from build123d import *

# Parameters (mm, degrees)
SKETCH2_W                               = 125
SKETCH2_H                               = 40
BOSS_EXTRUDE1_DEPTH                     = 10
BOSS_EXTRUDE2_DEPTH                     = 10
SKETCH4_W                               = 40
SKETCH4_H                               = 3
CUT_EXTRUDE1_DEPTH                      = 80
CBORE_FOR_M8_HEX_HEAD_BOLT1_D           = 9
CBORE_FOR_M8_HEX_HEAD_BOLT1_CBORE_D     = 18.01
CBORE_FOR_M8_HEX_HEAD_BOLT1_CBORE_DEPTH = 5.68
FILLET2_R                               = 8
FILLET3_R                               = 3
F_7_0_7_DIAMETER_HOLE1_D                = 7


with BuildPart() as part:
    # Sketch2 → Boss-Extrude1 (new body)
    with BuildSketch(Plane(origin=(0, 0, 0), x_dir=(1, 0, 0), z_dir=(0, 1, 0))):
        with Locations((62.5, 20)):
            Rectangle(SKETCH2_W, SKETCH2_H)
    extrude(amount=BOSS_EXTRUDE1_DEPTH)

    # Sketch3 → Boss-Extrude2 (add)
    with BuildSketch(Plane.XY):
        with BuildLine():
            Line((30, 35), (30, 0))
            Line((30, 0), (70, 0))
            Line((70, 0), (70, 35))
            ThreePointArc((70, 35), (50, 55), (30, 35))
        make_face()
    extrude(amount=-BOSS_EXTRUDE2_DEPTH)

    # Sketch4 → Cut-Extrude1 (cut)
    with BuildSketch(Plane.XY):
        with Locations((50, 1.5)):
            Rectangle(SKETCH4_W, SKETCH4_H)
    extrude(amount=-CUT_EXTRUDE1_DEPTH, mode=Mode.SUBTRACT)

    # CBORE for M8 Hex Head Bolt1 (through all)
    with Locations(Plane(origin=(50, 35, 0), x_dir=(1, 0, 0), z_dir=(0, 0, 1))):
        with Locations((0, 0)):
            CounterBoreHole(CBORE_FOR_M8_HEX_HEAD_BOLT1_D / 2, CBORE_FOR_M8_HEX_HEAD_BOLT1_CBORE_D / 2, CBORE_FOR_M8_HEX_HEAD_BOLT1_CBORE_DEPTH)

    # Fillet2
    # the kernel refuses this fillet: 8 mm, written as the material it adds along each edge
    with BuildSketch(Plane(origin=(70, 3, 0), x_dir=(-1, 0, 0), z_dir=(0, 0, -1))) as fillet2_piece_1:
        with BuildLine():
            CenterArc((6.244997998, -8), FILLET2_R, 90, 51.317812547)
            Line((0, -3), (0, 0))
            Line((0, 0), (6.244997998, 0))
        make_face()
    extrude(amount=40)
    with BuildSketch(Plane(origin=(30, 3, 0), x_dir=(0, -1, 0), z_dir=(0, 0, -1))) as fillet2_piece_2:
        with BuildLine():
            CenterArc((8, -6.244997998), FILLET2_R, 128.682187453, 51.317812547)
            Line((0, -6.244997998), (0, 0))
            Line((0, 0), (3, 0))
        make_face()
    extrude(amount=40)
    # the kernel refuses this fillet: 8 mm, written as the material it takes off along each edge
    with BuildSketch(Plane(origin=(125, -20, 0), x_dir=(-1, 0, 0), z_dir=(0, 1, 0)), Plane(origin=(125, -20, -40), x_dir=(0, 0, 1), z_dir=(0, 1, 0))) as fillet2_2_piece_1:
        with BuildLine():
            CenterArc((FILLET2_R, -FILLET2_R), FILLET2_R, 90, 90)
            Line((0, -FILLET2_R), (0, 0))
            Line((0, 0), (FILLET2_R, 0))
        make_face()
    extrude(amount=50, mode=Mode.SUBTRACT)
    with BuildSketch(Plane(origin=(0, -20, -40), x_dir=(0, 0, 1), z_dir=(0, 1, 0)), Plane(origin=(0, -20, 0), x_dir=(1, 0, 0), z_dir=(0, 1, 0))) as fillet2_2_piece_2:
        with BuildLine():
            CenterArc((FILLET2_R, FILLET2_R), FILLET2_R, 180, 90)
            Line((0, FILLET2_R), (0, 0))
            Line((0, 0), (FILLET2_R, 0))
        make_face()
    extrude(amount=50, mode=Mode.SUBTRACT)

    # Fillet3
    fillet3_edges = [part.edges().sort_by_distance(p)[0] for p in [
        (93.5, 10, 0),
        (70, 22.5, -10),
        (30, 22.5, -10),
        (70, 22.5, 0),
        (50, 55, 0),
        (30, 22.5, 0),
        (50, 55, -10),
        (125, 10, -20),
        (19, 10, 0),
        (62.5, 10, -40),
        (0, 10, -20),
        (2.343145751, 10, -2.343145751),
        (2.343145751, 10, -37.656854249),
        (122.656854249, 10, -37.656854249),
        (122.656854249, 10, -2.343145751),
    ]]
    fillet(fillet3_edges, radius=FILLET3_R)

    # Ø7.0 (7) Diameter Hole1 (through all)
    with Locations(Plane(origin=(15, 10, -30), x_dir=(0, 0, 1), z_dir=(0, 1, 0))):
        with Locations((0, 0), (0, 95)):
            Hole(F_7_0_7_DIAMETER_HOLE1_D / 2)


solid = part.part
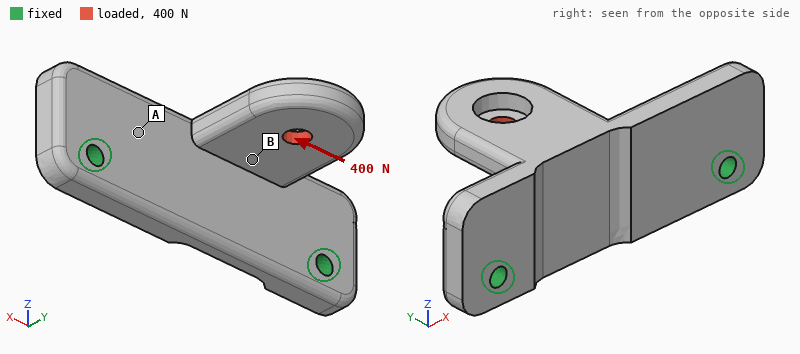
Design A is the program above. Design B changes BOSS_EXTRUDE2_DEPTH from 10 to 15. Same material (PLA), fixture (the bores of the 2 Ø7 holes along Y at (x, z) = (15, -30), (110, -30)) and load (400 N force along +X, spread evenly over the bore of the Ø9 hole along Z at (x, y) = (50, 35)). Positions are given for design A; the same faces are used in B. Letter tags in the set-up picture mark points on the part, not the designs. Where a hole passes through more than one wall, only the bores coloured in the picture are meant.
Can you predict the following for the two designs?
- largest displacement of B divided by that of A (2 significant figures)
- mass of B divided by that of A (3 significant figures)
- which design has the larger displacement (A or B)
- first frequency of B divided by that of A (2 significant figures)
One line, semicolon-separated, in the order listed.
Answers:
0.72; 1.14; A; 0.94
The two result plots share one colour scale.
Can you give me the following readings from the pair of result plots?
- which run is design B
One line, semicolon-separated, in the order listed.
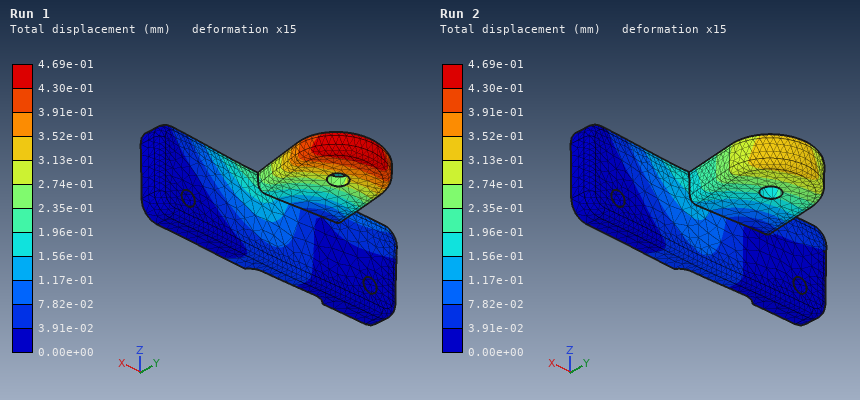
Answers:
Run 2
